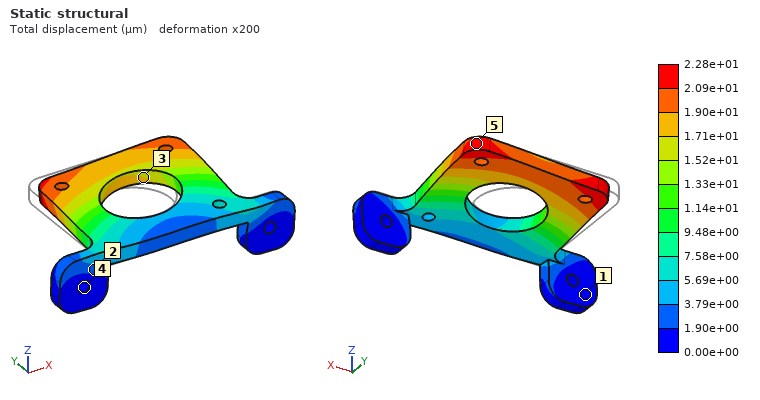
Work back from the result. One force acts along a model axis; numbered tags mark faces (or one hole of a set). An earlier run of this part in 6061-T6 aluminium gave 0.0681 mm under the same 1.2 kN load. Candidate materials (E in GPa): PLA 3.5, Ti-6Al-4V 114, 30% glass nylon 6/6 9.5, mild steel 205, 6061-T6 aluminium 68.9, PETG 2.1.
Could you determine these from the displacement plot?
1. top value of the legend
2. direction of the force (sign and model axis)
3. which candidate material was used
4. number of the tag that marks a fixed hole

2.28e+01 µm
+X
mild steel
4
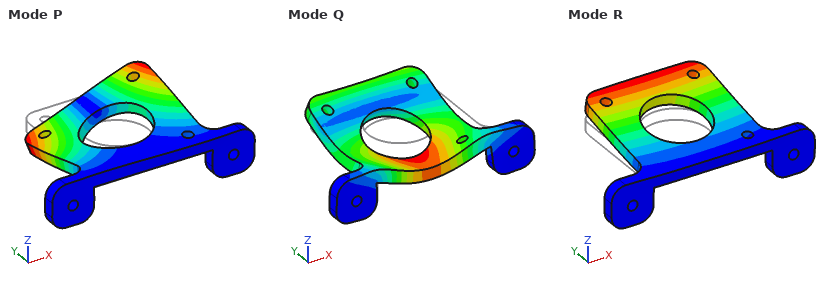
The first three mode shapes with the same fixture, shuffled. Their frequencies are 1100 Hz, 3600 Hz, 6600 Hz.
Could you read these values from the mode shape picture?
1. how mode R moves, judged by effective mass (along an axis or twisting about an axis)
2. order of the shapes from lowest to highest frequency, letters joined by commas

along Z
R, P, Q
